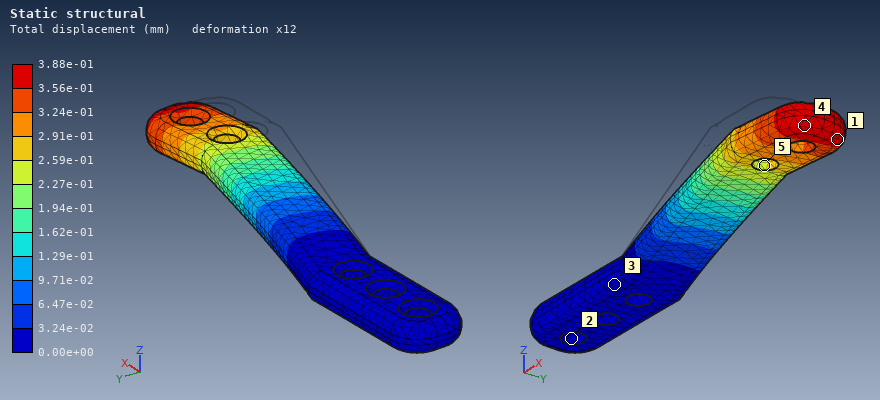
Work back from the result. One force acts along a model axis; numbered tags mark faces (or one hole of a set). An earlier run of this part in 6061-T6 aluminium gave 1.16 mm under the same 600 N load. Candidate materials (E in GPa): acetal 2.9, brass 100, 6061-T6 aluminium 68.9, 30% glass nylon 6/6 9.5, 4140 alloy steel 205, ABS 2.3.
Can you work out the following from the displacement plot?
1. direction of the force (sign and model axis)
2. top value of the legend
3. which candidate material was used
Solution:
+Y
3.88e-01 mm
4140 alloy steel
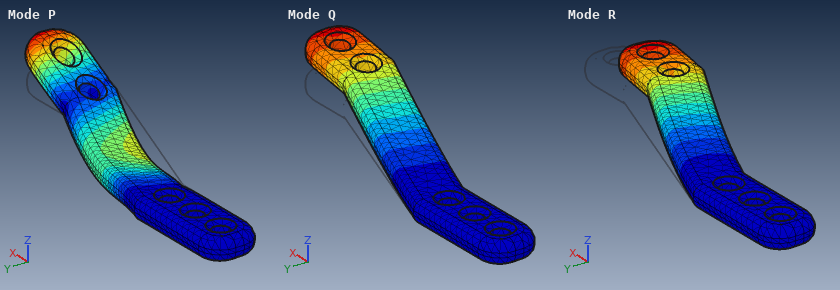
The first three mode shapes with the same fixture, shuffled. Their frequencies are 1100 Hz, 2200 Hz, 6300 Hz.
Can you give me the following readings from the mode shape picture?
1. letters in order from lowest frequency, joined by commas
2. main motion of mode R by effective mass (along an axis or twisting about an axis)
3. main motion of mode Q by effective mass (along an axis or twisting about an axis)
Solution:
Q, R, P
along Y
along Z
